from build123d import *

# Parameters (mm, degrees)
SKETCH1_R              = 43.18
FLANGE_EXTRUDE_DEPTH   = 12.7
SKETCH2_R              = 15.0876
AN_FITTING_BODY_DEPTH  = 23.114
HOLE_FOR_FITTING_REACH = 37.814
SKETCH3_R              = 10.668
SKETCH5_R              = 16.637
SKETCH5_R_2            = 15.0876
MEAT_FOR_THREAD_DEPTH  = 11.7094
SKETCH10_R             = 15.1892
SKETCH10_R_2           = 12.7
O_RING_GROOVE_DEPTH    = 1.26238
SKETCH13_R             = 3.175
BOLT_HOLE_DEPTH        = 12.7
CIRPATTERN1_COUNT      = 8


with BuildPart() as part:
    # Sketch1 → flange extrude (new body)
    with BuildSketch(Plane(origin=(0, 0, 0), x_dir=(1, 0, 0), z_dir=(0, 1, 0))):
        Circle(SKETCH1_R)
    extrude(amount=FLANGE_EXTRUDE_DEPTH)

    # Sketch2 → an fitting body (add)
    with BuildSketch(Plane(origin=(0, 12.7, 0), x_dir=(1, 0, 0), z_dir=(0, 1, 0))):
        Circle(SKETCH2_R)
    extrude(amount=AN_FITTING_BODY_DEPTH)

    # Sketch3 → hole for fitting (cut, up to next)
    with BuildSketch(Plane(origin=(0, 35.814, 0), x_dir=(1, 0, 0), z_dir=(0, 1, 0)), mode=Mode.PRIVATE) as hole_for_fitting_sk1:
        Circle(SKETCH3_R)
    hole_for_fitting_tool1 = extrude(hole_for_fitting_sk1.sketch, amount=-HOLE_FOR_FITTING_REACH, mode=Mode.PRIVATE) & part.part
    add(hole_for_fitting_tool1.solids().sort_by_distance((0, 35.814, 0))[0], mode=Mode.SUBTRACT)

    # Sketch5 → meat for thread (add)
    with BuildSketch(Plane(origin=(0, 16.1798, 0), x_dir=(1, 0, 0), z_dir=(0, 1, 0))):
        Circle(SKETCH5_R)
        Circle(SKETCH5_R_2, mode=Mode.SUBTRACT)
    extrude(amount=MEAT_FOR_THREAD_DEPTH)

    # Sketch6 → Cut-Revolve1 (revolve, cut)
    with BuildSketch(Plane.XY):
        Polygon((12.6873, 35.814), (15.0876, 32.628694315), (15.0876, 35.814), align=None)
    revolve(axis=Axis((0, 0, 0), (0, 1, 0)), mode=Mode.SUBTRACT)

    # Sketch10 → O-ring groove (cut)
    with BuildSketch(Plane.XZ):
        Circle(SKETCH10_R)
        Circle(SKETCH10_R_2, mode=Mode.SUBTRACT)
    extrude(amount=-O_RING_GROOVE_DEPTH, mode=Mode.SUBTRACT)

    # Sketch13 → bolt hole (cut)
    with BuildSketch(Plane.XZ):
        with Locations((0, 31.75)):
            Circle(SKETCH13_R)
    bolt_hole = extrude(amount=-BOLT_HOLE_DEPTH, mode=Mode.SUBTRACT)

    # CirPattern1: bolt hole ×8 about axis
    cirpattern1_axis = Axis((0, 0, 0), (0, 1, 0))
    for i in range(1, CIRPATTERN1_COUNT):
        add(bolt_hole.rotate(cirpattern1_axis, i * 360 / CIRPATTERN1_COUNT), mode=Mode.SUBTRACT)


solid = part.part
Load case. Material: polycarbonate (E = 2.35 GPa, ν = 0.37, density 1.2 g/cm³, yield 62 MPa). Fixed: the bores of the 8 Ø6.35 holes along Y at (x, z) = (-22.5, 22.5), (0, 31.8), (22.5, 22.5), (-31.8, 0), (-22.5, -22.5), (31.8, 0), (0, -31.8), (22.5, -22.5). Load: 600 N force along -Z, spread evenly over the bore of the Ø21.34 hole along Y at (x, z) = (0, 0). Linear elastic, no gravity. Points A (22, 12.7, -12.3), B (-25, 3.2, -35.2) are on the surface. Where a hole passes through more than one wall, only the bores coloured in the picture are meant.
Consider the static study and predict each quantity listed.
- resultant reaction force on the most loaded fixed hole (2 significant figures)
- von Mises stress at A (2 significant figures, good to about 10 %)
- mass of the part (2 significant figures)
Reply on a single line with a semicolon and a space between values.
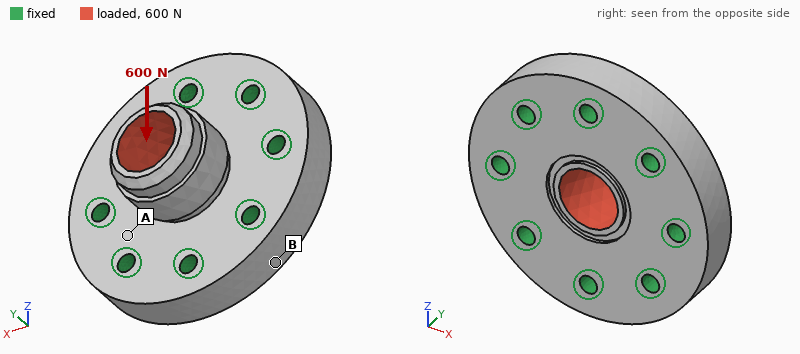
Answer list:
150 N; 0.51 MPa; 91 g
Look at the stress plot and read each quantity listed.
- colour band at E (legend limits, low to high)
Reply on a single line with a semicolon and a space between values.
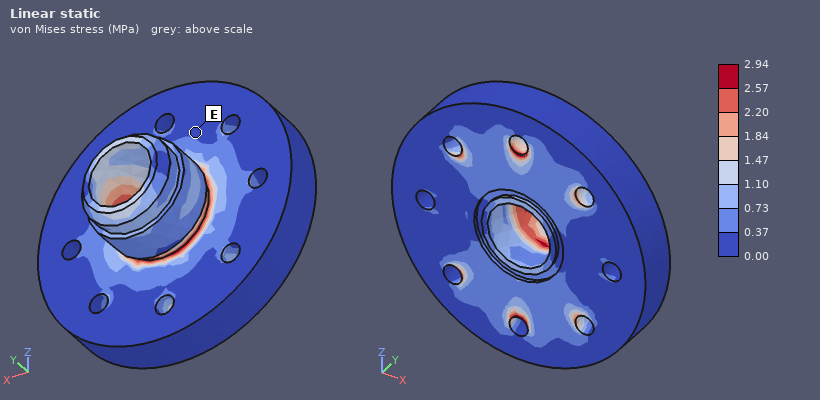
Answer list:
0.00 to 0.37 MPa
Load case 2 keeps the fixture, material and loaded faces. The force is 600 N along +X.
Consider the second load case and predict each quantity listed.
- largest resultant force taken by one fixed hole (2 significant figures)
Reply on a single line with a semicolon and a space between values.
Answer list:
150 N
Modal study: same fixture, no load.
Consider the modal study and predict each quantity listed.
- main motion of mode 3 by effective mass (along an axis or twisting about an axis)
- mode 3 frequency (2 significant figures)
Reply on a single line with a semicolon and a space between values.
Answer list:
along Y; 5500 Hz
